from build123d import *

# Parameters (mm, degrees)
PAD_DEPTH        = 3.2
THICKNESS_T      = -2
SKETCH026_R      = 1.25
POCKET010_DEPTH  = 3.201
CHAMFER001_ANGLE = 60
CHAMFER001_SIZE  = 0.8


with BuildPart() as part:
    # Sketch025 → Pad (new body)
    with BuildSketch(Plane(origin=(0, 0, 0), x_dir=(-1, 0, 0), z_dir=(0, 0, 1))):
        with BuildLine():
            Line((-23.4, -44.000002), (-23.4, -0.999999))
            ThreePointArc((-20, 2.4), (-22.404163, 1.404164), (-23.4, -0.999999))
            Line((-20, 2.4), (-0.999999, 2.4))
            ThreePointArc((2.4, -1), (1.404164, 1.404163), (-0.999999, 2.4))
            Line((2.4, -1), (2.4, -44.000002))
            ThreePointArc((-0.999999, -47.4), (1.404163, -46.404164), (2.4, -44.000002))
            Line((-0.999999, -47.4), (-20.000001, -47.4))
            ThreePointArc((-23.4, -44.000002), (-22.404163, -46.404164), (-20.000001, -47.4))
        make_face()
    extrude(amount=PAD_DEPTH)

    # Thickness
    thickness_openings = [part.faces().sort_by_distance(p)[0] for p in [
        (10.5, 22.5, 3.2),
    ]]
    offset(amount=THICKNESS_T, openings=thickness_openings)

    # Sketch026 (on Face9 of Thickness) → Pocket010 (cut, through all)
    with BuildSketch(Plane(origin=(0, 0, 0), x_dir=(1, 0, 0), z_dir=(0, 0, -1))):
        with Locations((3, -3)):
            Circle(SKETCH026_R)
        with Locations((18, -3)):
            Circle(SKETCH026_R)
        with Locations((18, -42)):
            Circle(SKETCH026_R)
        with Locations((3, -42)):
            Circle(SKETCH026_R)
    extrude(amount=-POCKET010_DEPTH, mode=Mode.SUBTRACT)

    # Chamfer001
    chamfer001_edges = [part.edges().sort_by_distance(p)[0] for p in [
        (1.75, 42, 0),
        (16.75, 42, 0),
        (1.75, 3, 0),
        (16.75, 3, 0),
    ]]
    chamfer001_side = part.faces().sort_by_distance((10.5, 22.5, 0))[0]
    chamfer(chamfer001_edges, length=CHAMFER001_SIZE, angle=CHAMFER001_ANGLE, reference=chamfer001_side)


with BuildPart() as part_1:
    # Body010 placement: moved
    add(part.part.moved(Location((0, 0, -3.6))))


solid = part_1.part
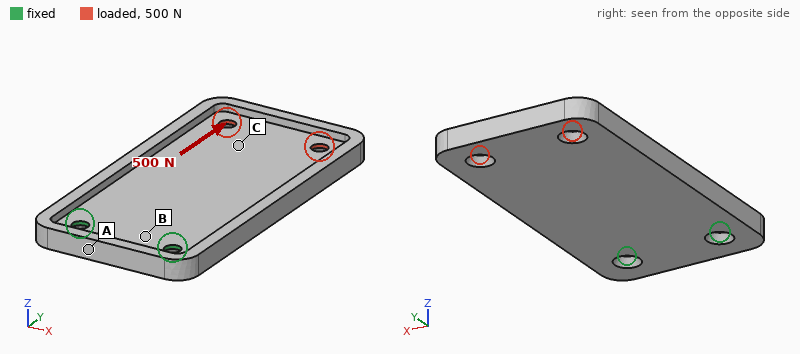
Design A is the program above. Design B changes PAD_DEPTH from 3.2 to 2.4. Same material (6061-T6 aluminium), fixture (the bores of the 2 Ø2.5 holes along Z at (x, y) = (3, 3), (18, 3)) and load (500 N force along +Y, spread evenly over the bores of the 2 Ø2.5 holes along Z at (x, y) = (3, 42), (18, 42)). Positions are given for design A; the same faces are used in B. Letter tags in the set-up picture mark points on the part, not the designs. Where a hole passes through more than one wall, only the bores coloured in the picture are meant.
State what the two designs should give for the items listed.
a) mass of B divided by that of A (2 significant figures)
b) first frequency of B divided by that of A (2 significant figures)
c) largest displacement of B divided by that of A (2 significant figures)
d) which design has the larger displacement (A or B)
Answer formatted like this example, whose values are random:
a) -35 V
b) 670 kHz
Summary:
a) 0.92
b) 0.95
c) 1.7
d) B
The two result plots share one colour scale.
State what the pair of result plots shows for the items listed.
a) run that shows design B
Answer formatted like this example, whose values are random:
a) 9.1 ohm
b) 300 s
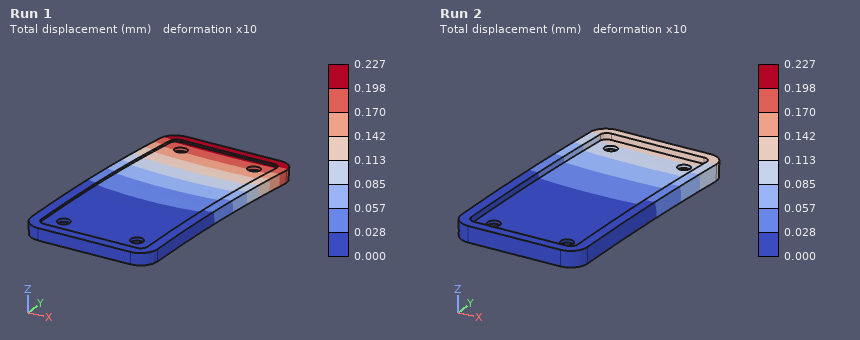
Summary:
a) Run 1
